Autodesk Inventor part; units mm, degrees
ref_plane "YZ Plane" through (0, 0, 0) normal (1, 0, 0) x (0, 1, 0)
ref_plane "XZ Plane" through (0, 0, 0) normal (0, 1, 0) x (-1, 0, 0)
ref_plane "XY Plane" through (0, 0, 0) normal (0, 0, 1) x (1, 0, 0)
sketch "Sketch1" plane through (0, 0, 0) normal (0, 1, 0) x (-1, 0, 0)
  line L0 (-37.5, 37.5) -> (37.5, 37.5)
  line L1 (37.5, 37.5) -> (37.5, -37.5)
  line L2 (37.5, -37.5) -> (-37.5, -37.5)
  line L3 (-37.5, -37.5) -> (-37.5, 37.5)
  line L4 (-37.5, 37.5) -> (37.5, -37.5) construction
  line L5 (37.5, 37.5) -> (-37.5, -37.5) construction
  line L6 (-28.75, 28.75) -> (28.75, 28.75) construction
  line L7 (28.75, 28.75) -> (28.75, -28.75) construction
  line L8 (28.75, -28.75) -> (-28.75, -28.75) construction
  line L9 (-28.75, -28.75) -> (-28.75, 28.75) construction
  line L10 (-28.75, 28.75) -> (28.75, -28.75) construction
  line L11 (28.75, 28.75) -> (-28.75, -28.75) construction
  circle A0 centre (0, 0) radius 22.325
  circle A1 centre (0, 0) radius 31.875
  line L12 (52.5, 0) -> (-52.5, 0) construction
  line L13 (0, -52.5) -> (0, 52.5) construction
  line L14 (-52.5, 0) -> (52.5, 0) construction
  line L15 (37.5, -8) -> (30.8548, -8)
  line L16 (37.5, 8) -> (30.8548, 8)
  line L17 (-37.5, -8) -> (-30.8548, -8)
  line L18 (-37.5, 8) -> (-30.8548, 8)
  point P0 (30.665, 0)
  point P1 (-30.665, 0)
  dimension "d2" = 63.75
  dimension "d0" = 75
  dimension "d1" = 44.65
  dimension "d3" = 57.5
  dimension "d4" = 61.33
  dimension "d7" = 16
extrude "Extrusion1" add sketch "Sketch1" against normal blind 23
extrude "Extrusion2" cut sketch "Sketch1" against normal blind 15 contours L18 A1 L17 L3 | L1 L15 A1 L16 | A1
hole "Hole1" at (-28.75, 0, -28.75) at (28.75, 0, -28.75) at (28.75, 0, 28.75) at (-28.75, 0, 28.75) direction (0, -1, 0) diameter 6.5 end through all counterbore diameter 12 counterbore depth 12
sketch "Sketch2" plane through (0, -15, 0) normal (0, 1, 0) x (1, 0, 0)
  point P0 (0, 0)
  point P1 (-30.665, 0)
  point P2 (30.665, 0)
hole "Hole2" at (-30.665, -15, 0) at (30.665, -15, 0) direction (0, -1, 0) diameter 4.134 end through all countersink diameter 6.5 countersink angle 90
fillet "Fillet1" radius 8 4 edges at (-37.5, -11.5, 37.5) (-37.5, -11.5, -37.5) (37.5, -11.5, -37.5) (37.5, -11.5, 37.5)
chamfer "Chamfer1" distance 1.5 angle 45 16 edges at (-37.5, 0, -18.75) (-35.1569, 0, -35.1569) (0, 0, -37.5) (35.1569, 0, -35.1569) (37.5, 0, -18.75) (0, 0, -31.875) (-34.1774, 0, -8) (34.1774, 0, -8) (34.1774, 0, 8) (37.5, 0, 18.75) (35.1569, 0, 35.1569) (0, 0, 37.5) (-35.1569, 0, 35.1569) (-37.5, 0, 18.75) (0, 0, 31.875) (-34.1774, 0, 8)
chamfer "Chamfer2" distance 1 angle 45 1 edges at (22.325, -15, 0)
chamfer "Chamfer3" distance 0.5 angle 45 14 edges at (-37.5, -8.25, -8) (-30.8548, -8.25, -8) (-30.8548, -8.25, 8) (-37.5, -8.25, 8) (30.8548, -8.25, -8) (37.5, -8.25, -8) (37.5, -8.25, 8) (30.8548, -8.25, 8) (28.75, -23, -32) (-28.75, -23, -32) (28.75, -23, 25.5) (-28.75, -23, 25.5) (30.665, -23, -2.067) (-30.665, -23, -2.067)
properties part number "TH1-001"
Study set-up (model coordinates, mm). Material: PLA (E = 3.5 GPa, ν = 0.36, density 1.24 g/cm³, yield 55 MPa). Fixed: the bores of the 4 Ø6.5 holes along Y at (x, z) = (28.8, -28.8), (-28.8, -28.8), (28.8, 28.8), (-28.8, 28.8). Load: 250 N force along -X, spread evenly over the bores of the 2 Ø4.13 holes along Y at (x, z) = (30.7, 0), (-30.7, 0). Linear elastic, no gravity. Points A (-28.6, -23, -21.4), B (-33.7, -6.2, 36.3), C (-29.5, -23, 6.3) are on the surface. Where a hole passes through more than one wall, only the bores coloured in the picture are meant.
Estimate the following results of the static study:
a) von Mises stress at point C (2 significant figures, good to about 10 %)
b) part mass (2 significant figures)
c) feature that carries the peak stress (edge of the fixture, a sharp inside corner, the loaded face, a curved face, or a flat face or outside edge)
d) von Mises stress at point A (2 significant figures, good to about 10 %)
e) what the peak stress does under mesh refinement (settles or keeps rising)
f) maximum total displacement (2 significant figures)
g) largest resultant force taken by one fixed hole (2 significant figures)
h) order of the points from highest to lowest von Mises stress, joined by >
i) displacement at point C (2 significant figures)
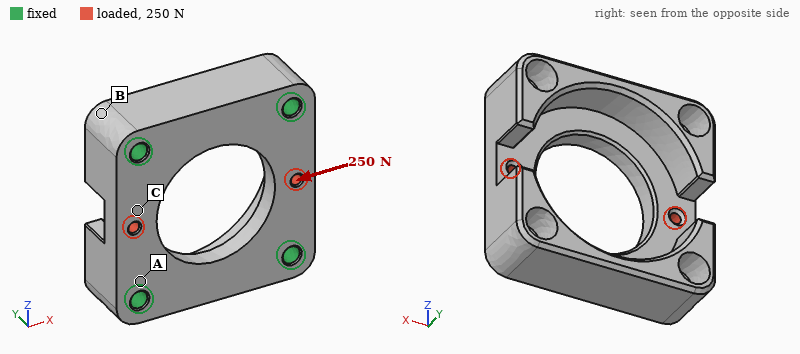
1.3 MPa
71 g
edge of the fixture
0.54 MPa
keeps rising
16 µm
63 N
C > A > B
12 µm
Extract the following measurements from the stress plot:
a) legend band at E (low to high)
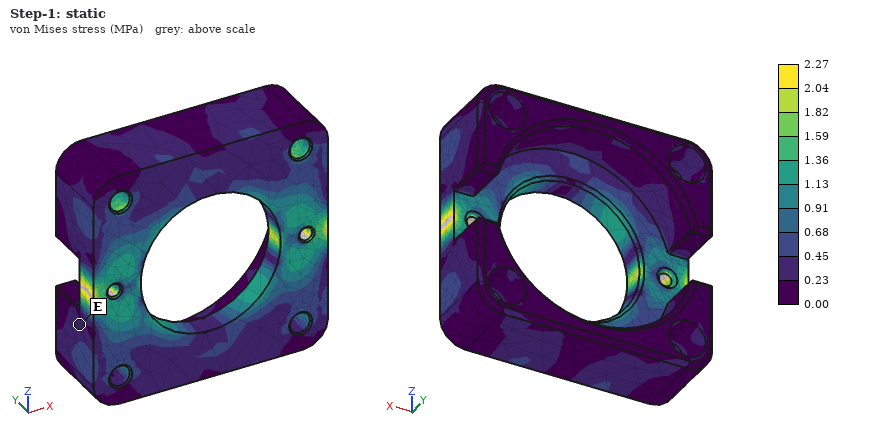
0.23 to 0.45 MPa
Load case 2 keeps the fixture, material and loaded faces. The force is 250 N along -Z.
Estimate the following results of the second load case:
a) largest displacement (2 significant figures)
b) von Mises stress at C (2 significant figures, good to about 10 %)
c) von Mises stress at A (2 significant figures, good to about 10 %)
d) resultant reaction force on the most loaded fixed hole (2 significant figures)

4.5 µm
0.77 MPa
0.47 MPa
63 N
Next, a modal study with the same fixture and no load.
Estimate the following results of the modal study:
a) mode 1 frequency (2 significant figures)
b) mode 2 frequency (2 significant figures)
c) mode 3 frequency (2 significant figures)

4000 Hz
4500 Hz
4700 Hz
